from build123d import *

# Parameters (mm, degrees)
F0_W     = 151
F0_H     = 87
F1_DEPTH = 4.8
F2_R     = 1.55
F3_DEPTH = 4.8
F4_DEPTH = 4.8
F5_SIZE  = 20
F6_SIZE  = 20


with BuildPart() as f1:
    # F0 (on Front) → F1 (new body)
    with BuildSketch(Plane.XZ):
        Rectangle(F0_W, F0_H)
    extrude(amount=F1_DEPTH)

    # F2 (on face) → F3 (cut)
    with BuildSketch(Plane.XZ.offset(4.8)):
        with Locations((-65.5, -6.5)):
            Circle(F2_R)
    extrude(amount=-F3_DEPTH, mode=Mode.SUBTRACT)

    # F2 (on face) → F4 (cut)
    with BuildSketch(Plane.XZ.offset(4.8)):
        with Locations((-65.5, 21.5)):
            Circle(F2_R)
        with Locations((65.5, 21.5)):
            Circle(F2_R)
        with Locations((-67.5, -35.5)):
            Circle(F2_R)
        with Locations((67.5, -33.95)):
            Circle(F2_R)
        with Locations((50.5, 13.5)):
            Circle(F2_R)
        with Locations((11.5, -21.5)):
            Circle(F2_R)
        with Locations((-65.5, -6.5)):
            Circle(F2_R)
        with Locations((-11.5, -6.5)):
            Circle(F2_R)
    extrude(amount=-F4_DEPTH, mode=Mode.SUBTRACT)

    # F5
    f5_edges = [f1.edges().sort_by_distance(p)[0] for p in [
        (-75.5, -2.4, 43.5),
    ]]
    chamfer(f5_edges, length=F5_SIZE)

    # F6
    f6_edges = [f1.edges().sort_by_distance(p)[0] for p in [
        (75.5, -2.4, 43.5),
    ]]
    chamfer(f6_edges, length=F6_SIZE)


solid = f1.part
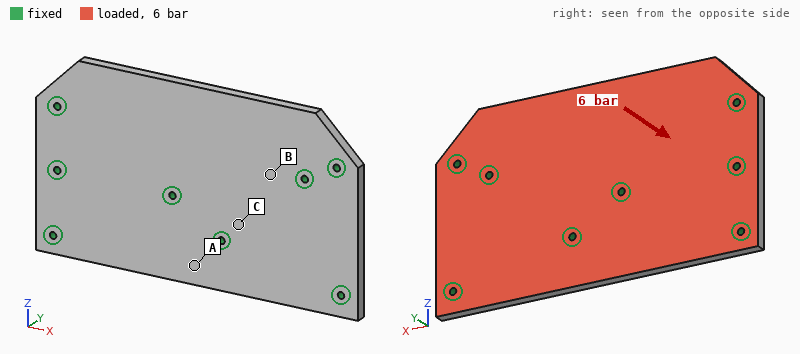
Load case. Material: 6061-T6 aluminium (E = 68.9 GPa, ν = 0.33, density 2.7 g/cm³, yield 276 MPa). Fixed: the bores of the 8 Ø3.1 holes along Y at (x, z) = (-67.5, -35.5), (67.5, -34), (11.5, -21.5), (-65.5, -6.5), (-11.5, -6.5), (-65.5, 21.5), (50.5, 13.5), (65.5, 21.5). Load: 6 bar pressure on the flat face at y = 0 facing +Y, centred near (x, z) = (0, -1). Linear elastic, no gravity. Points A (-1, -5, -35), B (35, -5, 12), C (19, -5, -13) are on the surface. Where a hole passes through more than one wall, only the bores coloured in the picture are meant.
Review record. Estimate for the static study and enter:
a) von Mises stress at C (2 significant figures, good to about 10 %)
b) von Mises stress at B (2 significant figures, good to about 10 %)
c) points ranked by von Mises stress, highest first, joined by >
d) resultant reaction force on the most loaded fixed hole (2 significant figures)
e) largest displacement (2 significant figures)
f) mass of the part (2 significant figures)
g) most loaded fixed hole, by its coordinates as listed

33 MPa
56 MPa
B > C > A
2.1 kN
0.42 mm
160 g
(-11.5, -6.5)
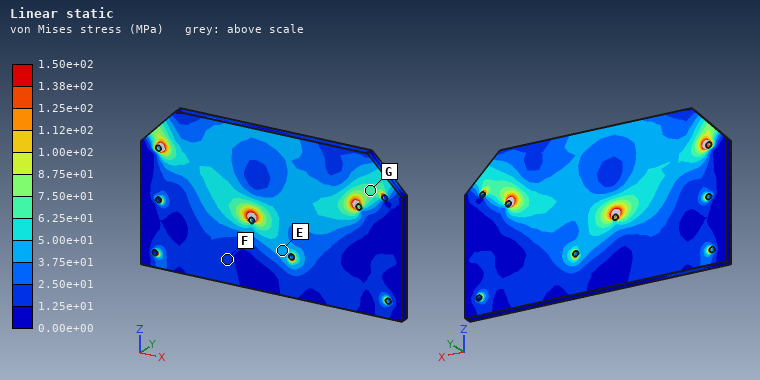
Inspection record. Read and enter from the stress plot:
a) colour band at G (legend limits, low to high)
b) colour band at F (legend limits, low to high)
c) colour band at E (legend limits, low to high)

6.25e+01 to 7.50e+01 MPa
1.25e+01 to 2.50e+01 MPa
3.75e+01 to 5.00e+01 MPa
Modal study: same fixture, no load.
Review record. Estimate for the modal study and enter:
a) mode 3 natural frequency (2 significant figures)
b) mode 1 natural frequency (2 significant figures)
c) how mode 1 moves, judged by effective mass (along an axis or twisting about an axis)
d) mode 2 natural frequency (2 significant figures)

4400 Hz
2200 Hz
along Y
4300 Hz
